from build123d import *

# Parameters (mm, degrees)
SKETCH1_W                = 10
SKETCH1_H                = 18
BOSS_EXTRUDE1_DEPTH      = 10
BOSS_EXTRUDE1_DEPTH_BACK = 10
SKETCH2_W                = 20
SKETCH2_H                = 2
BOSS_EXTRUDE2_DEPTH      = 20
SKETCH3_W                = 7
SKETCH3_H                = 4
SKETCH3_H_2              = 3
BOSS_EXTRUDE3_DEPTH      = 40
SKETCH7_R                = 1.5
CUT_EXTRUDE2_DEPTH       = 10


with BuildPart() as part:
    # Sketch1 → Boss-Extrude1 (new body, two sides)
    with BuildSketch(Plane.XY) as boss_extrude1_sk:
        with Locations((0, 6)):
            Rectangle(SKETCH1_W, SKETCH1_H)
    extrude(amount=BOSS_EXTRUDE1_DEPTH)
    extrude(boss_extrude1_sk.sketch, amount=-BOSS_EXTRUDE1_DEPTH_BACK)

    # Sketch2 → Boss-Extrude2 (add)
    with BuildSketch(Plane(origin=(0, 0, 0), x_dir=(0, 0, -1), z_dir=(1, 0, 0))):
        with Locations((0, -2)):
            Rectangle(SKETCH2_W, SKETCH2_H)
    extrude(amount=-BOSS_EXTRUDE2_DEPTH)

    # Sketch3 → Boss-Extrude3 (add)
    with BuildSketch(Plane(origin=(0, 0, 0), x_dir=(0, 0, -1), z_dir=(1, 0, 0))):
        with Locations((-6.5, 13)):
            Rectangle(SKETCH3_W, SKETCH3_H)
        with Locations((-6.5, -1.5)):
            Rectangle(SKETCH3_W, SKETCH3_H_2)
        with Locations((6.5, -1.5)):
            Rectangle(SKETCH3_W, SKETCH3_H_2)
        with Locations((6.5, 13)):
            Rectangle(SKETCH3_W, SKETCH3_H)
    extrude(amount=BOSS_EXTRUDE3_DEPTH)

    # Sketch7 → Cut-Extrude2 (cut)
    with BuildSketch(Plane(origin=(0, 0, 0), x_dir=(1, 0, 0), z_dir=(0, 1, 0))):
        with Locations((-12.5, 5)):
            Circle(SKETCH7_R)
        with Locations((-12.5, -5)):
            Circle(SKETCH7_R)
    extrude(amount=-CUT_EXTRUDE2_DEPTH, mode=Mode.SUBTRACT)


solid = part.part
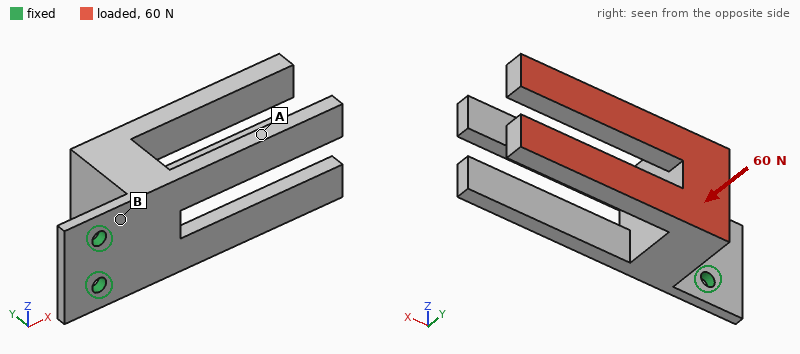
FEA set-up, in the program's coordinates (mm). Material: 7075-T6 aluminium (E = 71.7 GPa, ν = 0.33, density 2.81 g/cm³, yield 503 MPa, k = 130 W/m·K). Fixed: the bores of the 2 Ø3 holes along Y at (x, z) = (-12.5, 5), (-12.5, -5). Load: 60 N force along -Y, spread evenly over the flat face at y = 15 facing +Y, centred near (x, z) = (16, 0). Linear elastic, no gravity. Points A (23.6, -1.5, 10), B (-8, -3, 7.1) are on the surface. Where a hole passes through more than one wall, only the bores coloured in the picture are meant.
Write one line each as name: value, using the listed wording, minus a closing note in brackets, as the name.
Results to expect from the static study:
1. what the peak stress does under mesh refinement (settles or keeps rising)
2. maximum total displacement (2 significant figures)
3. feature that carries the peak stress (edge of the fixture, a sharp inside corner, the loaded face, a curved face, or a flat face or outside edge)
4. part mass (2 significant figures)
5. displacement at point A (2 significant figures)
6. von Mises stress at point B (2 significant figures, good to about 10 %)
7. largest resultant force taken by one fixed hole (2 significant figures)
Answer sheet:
what the peak stress does under mesh refinement: keeps rising
maximum total displacement: 0.62 mm
feature that carries the peak stress: edge of the fixture
part mass: 21 g
displacement at point A: 0.35 mm
von Mises stress at point B: 97 MPa
largest resultant force taken by one fixed hole: 30 N
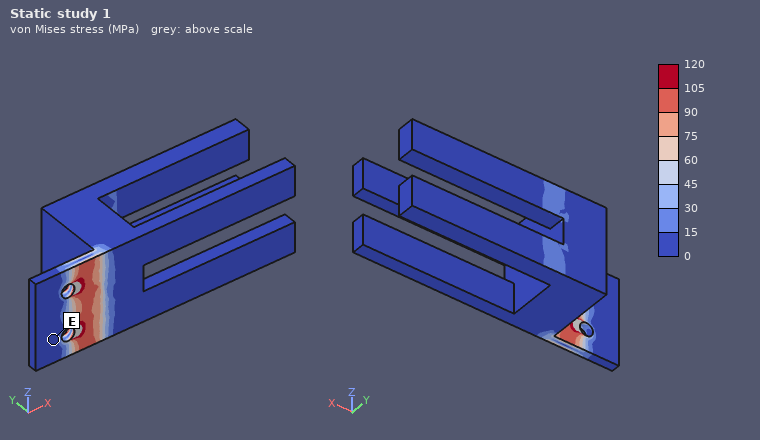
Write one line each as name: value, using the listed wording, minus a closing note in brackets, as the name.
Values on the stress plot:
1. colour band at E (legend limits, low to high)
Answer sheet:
colour band at E: 0 to 15 MPa
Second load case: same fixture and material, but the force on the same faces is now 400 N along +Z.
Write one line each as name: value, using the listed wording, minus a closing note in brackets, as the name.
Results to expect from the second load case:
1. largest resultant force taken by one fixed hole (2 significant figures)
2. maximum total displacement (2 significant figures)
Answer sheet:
largest resultant force taken by one fixed hole: 1.1 kN
maximum total displacement: 0.36 mm
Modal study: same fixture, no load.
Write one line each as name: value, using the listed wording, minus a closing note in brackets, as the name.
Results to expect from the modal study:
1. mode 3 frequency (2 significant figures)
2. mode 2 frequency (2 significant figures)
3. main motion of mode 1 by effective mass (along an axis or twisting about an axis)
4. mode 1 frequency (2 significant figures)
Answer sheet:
mode 3 frequency: 2000 Hz
mode 2 frequency: 1800 Hz
main motion of mode 1 by effective mass: along Y
mode 1 frequency: 500 Hz
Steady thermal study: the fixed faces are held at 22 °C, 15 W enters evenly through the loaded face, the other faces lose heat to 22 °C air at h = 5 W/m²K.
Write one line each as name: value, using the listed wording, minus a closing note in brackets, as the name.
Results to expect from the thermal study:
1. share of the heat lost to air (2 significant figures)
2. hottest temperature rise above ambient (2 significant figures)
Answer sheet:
share of the heat lost to air: 4.4 %
hottest temperature rise above ambient: 61 K
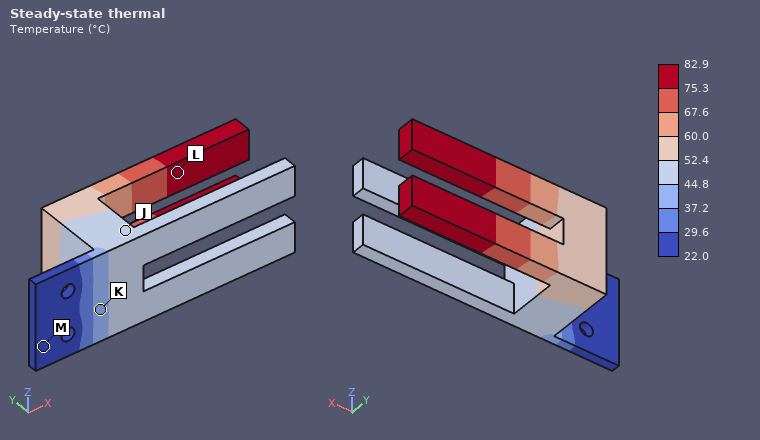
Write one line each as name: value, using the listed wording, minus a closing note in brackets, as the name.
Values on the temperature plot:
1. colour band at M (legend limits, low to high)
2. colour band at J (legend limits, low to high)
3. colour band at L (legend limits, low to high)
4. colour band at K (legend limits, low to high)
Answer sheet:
colour band at M: 22.0 to 29.6 °C
colour band at J: 44.8 to 52.4 °C
colour band at L: 75.3 to 82.9 °C
colour band at K: 37.2 to 44.8 °C
